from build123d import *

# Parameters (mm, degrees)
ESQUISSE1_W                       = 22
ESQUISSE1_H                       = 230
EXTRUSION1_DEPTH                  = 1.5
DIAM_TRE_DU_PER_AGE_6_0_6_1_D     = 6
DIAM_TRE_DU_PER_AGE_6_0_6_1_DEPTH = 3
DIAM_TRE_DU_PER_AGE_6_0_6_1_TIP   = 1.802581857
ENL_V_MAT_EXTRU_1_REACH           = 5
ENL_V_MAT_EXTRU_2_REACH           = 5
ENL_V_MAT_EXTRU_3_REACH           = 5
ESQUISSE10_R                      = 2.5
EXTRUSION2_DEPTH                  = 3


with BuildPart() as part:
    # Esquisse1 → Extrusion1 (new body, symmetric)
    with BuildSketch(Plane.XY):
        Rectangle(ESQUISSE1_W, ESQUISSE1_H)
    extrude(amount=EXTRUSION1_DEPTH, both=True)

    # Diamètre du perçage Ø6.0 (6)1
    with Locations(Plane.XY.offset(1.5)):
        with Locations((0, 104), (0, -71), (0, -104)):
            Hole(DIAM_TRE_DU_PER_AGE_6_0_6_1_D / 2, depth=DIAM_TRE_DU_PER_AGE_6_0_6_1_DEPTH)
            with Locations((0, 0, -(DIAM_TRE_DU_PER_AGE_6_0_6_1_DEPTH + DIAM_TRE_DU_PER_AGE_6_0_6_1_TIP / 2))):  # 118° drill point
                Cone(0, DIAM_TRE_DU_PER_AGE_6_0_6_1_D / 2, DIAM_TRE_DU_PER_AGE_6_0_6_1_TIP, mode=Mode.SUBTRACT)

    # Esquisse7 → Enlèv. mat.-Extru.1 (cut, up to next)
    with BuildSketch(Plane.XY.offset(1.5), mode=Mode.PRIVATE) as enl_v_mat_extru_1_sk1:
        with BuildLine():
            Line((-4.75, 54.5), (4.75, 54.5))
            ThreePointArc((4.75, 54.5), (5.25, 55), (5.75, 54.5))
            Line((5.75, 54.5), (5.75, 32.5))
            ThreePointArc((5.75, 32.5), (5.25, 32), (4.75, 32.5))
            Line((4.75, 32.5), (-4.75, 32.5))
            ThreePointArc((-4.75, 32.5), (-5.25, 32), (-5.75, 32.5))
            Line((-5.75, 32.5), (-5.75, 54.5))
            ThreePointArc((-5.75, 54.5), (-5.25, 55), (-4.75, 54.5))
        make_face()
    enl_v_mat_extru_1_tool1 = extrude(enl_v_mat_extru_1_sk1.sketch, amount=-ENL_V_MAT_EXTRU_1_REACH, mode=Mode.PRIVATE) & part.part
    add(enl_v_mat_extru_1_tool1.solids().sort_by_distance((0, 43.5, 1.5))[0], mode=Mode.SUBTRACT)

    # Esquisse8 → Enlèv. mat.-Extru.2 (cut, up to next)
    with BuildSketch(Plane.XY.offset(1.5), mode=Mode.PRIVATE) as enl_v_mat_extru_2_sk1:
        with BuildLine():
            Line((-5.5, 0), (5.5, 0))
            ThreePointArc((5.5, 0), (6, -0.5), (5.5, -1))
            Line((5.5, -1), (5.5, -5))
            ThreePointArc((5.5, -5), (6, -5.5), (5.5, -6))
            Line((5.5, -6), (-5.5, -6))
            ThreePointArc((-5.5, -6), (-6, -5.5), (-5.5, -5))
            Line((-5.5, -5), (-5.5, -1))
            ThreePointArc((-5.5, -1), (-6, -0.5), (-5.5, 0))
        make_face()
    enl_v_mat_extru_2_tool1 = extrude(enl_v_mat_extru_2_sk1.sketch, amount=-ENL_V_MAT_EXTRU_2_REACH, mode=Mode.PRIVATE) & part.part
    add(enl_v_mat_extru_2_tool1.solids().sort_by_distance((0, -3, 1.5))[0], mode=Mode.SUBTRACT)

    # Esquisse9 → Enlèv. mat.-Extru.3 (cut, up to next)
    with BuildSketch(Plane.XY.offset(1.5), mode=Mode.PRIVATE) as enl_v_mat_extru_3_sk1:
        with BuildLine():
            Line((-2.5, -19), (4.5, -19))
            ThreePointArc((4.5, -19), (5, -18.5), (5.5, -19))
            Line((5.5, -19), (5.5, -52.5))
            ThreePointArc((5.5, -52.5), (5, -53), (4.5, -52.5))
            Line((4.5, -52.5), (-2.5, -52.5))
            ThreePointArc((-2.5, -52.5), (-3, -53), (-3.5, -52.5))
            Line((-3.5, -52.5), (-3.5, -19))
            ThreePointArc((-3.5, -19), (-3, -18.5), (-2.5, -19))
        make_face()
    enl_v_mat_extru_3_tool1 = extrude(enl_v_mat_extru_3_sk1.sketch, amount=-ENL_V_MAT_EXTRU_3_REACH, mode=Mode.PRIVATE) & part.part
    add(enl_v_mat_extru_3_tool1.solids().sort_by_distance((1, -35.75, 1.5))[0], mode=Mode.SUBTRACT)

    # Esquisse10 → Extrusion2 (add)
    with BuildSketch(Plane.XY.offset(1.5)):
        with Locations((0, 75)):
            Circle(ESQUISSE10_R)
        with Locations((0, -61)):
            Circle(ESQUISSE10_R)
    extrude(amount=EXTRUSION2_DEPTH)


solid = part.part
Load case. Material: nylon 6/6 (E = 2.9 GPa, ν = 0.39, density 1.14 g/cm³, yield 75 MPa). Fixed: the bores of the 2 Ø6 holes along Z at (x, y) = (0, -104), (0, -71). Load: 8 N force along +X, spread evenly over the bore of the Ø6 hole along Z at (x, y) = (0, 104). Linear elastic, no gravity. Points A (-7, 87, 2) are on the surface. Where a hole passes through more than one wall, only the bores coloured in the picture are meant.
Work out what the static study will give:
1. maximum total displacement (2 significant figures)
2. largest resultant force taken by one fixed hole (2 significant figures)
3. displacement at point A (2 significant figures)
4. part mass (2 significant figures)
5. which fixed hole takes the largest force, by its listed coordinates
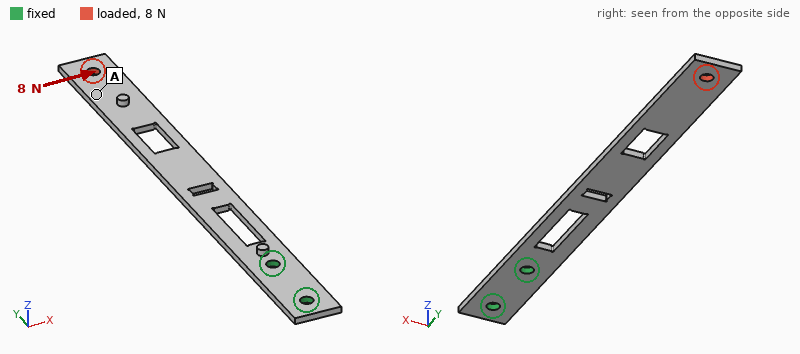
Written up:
2.7 mm
33 N
2.1 mm
15 g
(0, -71)
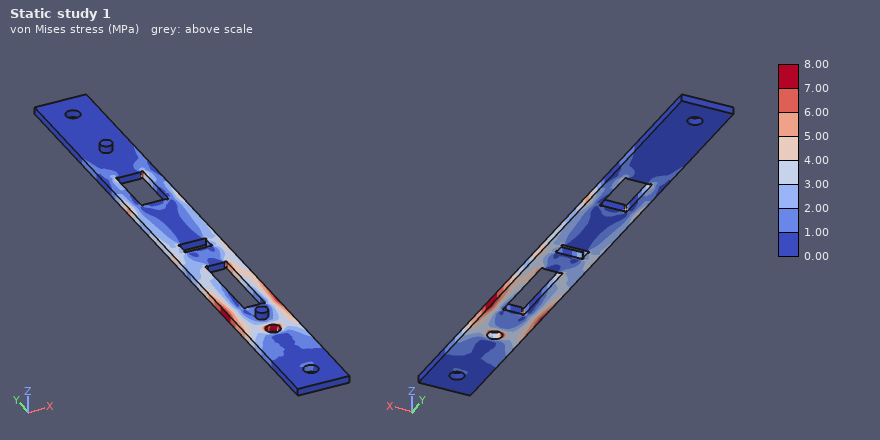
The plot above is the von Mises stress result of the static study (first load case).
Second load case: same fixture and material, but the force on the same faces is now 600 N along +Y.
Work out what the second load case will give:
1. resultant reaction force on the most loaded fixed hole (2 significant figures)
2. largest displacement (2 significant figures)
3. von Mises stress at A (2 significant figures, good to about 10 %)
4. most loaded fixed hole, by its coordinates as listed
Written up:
540 N
0.94 mm
9.1 MPa
(0, -71)
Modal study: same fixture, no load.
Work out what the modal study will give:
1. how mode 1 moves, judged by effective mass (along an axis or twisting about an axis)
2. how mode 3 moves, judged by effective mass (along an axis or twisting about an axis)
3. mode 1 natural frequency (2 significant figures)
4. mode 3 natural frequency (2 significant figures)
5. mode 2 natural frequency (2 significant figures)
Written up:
along Z
along X
20 Hz
140 Hz
130 Hz
